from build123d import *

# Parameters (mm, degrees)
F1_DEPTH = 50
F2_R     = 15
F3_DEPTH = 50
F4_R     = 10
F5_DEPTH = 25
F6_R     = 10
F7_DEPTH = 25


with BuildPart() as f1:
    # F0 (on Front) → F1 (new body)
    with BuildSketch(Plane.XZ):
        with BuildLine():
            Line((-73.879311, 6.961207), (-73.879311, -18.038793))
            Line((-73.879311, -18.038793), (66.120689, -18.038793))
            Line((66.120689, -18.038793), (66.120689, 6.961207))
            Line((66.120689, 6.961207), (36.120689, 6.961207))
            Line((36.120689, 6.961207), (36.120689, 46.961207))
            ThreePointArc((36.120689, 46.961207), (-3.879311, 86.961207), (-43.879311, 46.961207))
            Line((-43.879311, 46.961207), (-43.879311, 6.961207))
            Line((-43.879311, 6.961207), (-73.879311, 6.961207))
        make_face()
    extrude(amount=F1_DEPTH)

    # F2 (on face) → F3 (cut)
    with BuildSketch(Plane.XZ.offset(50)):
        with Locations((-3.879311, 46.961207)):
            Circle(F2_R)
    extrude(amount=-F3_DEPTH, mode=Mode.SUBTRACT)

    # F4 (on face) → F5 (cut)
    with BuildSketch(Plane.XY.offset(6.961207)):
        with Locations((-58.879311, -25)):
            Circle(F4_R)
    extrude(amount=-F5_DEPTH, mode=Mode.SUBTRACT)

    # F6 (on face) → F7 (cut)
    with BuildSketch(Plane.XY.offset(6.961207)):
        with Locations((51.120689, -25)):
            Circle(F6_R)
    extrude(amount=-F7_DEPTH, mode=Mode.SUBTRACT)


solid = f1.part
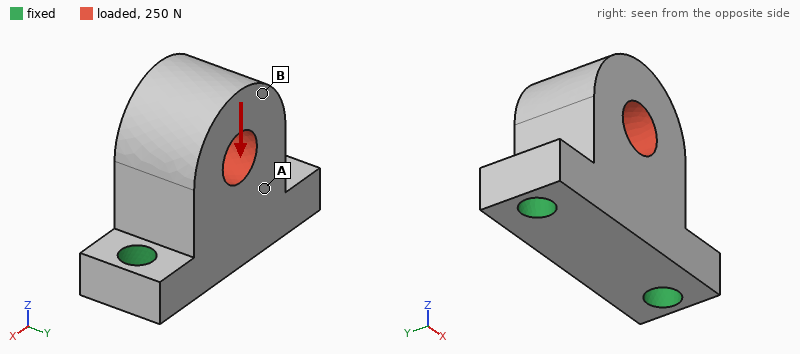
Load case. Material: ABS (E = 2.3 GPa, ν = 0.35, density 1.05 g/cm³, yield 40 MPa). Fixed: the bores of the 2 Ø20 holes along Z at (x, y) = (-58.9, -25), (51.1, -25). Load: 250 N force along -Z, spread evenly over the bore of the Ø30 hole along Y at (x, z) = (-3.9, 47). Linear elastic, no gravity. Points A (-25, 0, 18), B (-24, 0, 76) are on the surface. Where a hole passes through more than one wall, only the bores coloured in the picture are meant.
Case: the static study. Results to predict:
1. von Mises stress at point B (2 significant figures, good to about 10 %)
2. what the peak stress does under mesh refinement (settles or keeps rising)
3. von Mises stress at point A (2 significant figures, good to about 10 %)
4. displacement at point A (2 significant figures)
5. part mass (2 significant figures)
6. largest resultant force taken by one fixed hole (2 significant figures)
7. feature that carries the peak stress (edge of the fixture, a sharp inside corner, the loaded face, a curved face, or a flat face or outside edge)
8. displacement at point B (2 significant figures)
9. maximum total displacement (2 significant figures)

0.039 MPa
keeps rising
0.080 MPa
3.8 µm
430 g
130 N
edge of the fixture
5.0 µm
5.7 µm
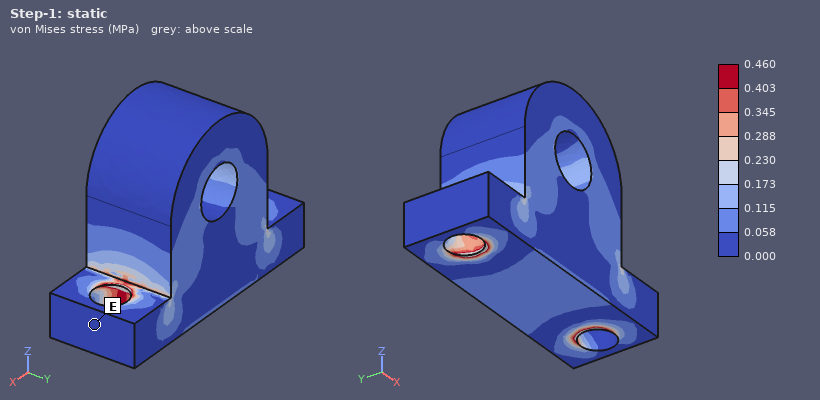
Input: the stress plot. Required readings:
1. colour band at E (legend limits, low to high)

0.000 to 0.058 MPa
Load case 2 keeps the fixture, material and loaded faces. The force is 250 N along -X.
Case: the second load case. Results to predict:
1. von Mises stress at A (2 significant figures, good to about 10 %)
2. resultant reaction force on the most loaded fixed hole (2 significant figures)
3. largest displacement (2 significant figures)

0.11 MPa
190 N
16 µm
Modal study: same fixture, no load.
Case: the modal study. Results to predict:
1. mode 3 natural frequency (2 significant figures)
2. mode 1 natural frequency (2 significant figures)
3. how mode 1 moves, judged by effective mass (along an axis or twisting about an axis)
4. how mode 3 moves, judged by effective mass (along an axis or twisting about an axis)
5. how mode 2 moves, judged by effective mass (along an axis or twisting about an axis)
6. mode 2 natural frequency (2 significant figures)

2100 Hz
680 Hz
along Y
along Z
along X
1500 Hz
